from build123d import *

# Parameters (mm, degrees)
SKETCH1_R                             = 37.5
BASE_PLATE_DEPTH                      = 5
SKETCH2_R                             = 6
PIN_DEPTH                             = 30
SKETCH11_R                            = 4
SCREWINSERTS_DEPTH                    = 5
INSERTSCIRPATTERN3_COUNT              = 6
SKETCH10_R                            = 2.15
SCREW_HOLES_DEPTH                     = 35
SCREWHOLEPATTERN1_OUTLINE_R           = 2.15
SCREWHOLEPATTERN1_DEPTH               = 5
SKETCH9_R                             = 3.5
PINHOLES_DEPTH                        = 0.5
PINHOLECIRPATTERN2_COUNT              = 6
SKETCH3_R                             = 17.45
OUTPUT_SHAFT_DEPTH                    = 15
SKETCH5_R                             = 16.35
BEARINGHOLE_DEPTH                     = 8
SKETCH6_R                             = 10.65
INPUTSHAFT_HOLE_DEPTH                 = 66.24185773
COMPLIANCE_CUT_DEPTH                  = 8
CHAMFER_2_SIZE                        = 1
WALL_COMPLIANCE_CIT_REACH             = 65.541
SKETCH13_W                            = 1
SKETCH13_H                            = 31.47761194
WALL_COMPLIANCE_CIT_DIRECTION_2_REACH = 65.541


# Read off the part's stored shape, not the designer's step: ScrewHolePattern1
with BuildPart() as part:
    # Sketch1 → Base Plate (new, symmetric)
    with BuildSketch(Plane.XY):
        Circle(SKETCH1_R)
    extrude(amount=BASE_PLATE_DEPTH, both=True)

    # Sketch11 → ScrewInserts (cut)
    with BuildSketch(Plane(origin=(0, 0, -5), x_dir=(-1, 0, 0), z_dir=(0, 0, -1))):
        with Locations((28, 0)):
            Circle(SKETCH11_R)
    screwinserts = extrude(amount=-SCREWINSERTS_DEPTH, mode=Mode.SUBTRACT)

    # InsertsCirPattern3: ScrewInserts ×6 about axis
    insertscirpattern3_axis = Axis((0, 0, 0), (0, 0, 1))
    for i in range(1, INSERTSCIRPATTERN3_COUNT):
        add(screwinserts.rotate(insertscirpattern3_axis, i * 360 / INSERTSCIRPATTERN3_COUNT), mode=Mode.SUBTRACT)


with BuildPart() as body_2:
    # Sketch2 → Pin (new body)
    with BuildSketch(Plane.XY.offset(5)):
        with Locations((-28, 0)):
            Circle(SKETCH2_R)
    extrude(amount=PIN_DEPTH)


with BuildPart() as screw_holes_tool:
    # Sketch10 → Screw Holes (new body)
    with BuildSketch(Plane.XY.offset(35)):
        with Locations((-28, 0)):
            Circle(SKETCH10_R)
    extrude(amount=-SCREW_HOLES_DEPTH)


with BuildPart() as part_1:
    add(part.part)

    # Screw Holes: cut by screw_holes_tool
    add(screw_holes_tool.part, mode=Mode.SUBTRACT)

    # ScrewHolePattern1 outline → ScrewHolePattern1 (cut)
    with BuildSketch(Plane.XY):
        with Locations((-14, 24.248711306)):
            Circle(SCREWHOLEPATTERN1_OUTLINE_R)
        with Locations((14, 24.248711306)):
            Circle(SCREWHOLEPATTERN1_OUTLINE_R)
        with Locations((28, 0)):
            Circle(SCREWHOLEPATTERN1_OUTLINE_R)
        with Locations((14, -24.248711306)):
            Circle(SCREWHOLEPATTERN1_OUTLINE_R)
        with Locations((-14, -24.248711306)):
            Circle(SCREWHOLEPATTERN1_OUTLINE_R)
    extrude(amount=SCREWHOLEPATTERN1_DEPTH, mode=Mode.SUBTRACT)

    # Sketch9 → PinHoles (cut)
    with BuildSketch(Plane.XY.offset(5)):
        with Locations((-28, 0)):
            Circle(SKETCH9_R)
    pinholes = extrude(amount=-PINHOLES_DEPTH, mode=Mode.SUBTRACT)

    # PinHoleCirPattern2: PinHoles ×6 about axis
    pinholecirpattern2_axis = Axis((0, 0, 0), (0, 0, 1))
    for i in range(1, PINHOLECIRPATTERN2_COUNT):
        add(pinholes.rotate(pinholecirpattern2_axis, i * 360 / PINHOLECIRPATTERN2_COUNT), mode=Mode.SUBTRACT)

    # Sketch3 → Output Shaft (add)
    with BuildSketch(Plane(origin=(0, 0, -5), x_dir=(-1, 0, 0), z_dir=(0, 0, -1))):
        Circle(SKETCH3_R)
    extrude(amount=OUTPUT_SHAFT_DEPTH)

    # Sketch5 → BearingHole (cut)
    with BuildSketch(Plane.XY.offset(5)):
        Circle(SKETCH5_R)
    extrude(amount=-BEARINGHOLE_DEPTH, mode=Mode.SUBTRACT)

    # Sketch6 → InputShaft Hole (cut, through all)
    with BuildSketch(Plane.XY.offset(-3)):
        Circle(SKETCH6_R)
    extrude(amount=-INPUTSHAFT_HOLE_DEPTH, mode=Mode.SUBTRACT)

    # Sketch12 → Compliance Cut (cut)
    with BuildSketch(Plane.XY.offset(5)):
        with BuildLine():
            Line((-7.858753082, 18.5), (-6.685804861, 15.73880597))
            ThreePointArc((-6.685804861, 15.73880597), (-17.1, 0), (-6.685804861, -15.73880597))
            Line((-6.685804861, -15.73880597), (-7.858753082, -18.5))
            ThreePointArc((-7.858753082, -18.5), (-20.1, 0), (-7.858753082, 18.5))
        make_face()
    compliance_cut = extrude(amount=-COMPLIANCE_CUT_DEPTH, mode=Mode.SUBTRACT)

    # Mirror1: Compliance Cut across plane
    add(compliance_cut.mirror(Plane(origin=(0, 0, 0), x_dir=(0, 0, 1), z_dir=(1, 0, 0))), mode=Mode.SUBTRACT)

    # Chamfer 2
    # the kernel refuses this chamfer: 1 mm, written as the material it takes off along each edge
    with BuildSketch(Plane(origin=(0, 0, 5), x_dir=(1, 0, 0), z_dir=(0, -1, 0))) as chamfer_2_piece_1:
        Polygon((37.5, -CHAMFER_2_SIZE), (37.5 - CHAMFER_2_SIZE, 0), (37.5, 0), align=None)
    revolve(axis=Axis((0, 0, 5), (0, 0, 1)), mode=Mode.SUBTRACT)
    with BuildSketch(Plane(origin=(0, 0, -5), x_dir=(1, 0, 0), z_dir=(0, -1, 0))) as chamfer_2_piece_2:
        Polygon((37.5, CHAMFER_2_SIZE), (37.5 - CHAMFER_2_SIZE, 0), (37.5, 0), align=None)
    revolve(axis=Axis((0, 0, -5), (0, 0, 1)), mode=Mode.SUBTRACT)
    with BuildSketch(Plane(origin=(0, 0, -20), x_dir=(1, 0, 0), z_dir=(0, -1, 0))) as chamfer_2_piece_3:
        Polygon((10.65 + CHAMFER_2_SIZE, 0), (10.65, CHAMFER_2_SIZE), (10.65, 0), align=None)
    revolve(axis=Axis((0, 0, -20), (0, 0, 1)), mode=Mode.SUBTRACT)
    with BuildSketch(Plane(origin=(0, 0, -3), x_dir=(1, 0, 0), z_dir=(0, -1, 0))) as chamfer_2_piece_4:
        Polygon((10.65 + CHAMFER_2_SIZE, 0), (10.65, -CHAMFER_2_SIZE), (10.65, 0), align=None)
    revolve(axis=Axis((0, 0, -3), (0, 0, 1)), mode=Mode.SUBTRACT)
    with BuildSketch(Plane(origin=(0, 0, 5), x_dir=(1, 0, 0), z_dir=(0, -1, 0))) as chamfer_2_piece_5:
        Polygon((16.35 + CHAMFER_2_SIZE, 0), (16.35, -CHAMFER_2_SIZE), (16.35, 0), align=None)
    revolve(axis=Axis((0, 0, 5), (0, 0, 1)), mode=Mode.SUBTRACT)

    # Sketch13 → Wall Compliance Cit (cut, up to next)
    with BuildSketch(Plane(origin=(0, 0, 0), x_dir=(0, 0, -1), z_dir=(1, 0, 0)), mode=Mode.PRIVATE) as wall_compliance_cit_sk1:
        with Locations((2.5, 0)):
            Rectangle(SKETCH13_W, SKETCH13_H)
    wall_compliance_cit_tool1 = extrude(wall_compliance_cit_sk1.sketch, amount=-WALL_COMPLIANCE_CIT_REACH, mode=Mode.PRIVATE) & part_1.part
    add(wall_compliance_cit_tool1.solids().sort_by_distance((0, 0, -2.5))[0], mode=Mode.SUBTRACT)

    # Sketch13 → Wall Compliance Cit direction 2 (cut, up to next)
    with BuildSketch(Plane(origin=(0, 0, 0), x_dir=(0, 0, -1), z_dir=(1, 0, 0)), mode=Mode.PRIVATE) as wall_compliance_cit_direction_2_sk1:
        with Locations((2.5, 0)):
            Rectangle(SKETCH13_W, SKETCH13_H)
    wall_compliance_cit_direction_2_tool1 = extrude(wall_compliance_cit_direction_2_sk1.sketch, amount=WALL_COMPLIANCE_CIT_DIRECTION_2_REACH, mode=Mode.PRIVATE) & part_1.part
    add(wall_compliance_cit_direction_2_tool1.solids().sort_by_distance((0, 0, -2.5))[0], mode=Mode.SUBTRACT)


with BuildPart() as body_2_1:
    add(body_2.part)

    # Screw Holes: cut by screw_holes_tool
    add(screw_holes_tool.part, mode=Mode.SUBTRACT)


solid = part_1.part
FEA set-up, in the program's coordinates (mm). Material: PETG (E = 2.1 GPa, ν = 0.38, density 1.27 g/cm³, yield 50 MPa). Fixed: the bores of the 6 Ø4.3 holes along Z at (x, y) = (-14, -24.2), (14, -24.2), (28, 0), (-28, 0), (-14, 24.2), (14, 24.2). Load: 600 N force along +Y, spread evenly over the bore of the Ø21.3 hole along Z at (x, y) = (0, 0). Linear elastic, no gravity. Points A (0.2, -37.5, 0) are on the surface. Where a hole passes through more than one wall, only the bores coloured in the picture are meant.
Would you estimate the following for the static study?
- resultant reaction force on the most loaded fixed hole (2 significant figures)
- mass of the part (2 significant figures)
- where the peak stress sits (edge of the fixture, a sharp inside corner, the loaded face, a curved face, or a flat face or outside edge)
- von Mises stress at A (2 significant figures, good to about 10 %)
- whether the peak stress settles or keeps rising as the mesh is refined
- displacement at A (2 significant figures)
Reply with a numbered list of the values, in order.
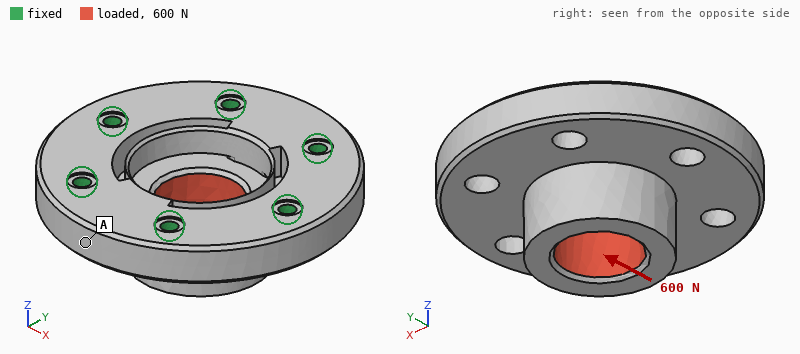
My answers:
1. 150 N
2. 52 g
3. edge of the fixture
4. 0.58 MPa
5. keeps rising
6. 16 µm
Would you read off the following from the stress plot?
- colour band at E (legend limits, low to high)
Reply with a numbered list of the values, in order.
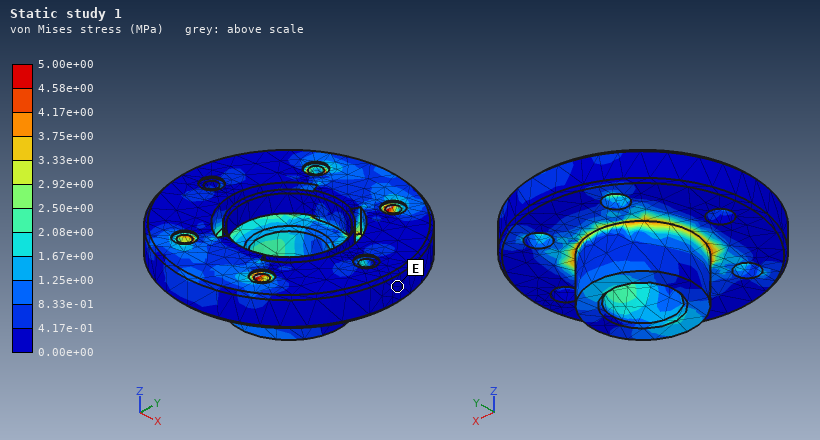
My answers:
1. 0.00e+00 to 4.17e-01 MPa
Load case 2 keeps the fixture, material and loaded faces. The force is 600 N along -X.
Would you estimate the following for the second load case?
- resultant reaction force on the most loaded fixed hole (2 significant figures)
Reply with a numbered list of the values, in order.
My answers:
1. 150 N
